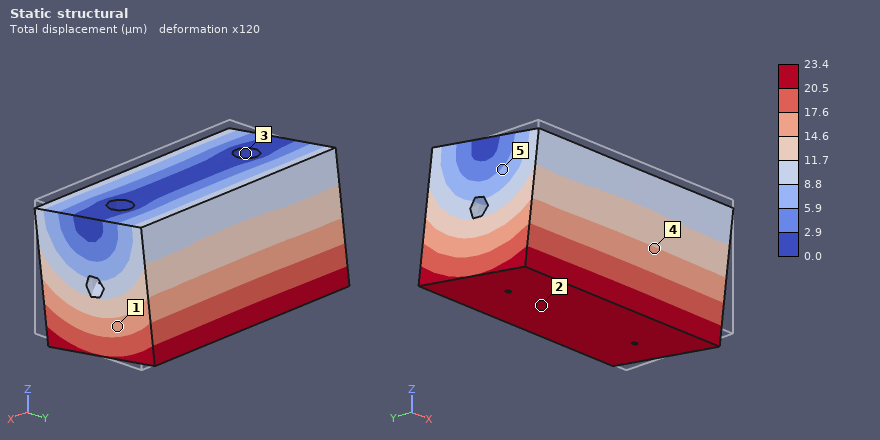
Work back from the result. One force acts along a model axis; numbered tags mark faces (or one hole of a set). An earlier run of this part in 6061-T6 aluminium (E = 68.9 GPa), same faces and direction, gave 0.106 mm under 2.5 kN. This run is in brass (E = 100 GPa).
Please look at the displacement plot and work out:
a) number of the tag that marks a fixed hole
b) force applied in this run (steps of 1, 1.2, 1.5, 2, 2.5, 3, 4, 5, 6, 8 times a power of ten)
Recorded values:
3
800 N
